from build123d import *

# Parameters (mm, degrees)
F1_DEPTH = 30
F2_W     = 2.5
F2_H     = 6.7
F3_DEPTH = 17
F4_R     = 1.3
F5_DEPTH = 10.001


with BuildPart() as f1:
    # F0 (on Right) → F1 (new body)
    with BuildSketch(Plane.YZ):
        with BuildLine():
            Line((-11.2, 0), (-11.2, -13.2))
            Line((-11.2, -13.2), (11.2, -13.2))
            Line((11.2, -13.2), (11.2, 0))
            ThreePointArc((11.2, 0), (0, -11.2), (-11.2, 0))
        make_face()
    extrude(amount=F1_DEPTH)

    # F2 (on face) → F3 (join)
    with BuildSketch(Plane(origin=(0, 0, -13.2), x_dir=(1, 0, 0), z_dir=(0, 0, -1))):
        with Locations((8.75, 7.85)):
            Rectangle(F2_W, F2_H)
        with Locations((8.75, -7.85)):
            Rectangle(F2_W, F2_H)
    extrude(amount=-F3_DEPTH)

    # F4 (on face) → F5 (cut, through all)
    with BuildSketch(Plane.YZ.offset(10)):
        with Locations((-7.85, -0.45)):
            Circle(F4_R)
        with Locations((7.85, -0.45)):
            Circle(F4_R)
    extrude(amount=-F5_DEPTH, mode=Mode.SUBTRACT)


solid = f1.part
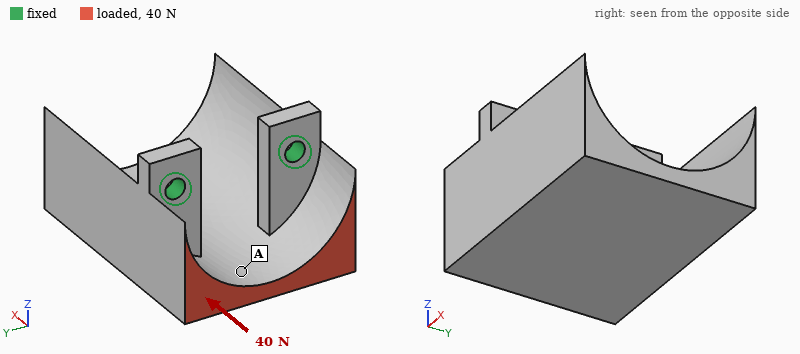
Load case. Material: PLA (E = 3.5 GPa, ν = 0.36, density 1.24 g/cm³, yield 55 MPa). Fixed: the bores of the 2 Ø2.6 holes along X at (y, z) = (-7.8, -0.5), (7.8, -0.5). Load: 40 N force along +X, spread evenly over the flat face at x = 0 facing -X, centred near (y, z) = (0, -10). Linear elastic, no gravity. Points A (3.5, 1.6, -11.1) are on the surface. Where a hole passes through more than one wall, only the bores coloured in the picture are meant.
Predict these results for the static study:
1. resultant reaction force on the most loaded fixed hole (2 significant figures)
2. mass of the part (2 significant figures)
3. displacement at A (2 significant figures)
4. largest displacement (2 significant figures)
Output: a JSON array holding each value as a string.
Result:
["20 N", "4.1 g", "0.17 mm", "0.39 mm"]
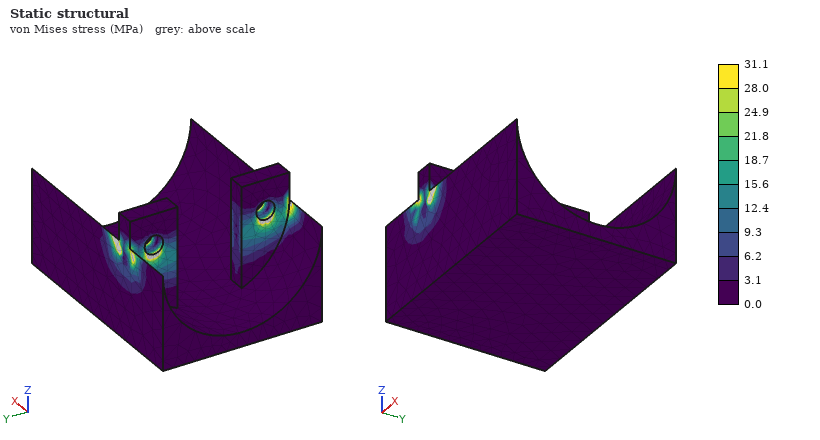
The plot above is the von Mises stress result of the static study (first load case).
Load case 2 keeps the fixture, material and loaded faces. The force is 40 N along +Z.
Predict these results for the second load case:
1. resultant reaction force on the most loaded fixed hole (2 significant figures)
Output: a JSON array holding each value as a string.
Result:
["20 N"]
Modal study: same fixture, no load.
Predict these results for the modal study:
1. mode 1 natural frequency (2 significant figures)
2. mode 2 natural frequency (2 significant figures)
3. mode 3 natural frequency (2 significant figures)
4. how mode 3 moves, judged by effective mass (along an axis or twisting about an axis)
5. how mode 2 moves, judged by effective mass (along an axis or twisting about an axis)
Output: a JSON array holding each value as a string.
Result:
["830 Hz", "1800 Hz", "3400 Hz", "along Y", "along Y"]
